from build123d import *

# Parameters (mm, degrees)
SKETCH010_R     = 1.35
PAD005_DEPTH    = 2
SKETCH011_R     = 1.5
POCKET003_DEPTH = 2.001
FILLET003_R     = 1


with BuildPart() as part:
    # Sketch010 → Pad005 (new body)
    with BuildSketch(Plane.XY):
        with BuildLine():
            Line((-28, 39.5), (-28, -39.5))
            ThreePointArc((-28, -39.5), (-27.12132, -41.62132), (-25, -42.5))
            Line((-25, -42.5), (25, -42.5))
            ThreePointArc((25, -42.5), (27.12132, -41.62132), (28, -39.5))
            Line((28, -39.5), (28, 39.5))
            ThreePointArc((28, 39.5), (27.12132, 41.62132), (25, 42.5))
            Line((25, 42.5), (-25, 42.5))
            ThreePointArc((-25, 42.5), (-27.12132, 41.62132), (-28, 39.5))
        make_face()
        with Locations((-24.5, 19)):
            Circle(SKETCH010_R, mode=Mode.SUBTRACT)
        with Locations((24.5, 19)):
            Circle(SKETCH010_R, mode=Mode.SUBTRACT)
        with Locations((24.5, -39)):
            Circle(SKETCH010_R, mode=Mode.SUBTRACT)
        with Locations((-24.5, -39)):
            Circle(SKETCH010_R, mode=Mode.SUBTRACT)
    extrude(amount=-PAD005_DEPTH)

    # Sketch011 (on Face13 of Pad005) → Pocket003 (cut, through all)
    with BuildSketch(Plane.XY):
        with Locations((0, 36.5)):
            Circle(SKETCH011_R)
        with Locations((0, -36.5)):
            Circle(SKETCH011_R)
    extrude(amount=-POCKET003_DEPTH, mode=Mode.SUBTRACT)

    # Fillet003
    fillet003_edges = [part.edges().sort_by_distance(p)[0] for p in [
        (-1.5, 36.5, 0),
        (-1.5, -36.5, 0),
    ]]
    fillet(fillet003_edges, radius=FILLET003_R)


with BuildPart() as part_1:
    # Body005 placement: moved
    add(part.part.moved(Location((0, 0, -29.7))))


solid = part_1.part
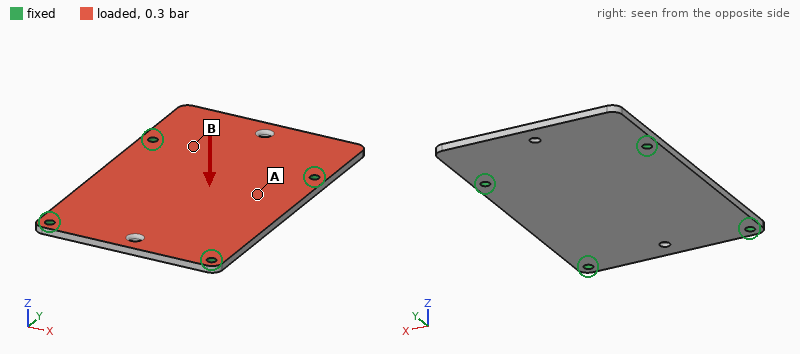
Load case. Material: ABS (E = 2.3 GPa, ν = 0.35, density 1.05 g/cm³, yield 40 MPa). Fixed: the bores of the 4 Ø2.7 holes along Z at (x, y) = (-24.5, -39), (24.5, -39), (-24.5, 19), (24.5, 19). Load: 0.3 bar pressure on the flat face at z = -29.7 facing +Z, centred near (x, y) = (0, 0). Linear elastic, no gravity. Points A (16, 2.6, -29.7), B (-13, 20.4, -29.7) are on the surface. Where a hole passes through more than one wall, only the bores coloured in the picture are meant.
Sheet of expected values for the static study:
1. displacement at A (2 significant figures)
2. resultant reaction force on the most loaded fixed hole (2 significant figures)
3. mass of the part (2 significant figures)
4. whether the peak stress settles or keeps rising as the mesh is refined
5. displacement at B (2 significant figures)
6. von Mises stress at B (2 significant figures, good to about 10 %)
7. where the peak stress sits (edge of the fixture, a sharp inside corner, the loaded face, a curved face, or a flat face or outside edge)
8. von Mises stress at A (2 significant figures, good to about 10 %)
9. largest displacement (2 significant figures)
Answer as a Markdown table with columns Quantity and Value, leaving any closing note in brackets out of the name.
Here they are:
| Quantity | Value |
|---|---|
| displacement at A | 0.65 mm |
| resultant reaction force on the most loaded fixed hole | 45 N |
| mass of the part | 9.9 g |
| whether the peak stress settles or keeps rising as the mesh is refined | keeps rising |
| displacement at B | 0.35 mm |
| von Mises stress at B | 9.0 MPa |
| where the peak stress sits | edge of the fixture |
| von Mises stress at A | 3.6 MPa |
| largest displacement | 1.2 mm |
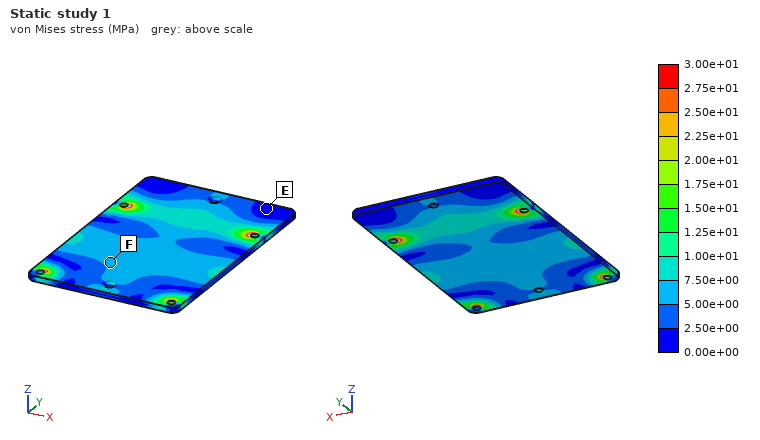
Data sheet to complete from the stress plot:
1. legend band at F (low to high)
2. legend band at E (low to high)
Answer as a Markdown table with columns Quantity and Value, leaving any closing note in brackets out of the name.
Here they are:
| Quantity | Value |
|---|---|
| legend band at F | 5.00e+00 to 7.50e+00 MPa |
| legend band at E | 0.00e+00 to 2.50e+00 MPa |
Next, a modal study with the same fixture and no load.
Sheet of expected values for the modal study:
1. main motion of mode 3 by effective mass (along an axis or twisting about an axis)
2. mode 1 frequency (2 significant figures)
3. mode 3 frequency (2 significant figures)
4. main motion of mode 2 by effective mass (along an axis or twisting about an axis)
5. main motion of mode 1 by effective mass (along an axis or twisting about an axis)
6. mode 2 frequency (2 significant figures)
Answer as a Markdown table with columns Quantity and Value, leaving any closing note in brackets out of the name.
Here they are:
| Quantity | Value |
|---|---|
| main motion of mode 3 by effective mass | twisting about Y |
| mode 1 frequency | 600 Hz |
| mode 3 frequency | 1100 Hz |
| main motion of mode 2 by effective mass | along Z |
| main motion of mode 1 by effective mass | twisting about X |
| mode 2 frequency | 710 Hz |
